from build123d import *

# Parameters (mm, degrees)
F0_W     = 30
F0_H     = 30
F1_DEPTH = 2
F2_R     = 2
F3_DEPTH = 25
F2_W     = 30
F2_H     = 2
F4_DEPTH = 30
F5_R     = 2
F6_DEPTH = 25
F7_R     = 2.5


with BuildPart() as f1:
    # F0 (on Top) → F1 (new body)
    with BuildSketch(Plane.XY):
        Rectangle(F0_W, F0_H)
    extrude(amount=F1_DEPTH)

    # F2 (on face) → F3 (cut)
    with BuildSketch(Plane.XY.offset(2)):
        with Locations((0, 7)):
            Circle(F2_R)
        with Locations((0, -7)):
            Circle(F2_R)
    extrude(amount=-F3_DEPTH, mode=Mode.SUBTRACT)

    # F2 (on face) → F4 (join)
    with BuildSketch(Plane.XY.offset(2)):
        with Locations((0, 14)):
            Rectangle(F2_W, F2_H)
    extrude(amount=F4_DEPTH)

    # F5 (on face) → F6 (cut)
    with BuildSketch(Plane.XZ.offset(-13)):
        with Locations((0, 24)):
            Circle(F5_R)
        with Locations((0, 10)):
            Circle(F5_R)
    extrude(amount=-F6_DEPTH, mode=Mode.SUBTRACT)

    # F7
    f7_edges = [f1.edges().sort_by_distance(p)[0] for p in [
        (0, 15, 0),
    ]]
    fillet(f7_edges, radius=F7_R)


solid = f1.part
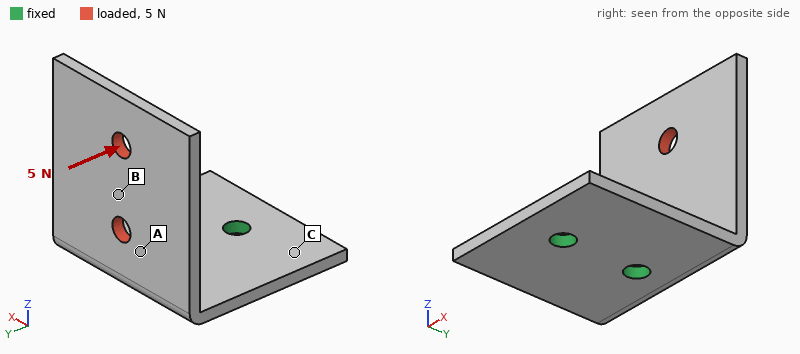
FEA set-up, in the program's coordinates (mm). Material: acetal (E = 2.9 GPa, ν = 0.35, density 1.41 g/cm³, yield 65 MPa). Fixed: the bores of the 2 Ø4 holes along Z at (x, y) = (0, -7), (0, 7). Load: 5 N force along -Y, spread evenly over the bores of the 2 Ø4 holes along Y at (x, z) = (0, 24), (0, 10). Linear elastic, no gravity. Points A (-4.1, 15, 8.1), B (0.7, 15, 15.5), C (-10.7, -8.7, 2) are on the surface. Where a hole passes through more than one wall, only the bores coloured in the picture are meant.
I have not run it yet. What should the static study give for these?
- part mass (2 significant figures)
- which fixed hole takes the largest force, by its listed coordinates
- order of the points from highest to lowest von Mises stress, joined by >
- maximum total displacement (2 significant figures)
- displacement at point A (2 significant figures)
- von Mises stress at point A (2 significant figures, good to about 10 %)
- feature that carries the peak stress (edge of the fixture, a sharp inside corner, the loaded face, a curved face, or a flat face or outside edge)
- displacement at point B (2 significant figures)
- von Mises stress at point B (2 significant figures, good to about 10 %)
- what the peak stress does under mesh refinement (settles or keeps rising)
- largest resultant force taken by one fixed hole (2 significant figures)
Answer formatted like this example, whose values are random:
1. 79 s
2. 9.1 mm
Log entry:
1. 4.9 g
2. (0, 7)
3. A > B > C
4. 0.61 mm
5. 0.11 mm
6. 2.3 MPa
7. edge of the fixture
8. 0.24 mm
9. 1.1 MPa
10. keeps rising
11. 4.6 N
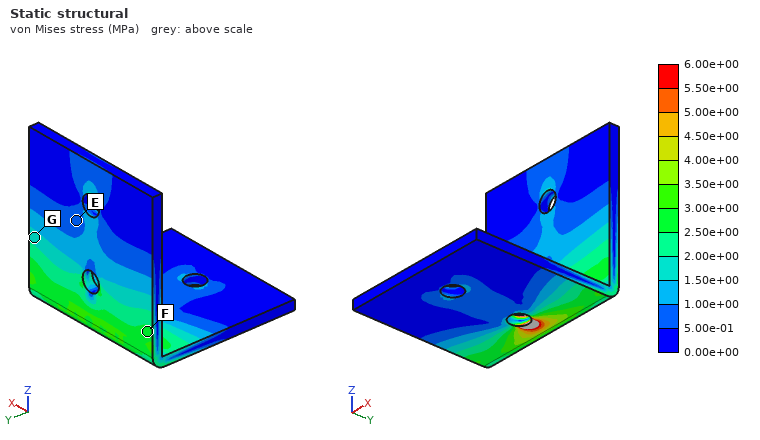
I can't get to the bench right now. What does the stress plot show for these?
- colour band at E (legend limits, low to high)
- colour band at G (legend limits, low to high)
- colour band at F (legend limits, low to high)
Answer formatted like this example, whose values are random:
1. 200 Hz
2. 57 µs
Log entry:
1. 5.00e-01 to 1.00e+00 MPa
2. 1.50e+00 to 2.00e+00 MPa
3. 2.50e+00 to 3.00e+00 MPa
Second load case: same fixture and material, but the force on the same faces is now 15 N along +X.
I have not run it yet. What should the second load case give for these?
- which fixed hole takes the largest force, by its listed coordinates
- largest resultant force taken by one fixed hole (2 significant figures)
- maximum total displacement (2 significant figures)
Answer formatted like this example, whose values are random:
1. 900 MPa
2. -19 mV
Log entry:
1. (0, 7)
2. 20 N
3. 0.55 mm
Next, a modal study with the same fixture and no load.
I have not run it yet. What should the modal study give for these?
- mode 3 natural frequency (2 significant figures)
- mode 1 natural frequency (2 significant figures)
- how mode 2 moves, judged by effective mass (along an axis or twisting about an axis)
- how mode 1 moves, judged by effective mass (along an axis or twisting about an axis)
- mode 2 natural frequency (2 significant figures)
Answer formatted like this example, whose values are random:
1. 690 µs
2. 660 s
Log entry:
1. 1100 Hz
2. 360 Hz
3. along X
4. along Y
5. 600 Hz
